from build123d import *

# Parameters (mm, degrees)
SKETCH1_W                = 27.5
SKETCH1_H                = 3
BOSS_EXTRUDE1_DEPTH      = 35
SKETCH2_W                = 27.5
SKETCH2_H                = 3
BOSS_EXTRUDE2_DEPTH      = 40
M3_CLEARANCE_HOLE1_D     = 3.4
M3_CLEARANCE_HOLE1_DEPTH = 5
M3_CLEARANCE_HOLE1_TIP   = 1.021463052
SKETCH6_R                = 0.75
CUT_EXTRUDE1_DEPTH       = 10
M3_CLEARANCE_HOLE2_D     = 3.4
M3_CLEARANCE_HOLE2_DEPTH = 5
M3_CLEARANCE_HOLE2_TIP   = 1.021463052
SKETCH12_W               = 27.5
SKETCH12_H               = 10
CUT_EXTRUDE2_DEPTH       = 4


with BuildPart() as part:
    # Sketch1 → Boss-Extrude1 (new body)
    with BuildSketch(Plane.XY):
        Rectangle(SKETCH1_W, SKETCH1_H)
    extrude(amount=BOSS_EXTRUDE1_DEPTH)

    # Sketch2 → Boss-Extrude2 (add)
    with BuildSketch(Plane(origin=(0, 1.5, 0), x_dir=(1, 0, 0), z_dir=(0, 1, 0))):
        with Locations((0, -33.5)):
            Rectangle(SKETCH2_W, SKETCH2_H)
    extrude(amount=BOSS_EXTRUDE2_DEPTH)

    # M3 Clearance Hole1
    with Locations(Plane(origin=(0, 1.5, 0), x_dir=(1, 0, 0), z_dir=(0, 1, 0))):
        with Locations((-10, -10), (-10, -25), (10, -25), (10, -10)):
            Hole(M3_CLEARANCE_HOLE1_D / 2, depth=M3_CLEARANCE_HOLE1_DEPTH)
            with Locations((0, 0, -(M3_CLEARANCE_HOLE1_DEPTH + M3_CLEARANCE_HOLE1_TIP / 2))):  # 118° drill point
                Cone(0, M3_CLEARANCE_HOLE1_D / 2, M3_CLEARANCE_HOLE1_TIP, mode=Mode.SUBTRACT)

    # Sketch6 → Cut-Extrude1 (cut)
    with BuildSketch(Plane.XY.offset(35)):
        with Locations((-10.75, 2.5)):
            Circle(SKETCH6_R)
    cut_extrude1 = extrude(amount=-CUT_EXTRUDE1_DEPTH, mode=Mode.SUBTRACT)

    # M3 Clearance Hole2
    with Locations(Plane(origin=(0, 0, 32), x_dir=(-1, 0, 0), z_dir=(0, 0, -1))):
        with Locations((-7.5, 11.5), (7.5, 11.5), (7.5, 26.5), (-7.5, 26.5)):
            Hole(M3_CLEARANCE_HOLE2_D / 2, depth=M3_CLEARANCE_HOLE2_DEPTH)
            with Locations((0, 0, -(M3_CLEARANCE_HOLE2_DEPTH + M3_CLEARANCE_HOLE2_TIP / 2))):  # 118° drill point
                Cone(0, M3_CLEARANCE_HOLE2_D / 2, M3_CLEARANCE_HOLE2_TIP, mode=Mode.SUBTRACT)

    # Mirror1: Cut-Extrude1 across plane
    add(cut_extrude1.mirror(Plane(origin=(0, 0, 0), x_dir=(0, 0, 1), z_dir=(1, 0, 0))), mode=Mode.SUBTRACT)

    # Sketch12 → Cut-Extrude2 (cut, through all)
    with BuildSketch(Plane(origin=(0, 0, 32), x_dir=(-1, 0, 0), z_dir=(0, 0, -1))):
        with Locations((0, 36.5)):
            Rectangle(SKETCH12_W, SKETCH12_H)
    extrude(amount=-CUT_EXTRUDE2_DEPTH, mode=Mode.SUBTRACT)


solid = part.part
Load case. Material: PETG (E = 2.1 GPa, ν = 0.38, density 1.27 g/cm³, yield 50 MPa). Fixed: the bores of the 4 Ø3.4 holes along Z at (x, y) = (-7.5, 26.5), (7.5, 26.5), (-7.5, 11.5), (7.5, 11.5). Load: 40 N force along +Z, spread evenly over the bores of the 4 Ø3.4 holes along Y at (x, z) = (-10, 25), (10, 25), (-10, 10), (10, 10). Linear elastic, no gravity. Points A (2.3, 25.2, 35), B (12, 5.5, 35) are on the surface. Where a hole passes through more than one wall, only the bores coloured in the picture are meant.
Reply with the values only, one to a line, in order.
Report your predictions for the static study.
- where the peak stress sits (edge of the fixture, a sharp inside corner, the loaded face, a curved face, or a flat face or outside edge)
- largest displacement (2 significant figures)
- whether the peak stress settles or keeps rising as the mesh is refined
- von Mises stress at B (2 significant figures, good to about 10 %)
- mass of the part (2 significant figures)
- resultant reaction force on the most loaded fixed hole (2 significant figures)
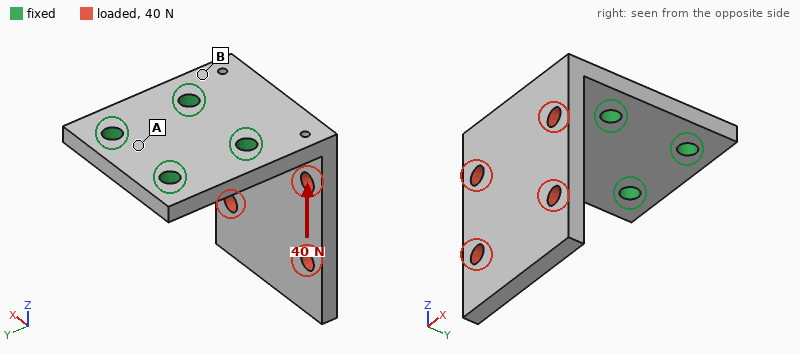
edge of the fixture
0.62 mm
keeps rising
4.9 MPa
6.5 g
23 N
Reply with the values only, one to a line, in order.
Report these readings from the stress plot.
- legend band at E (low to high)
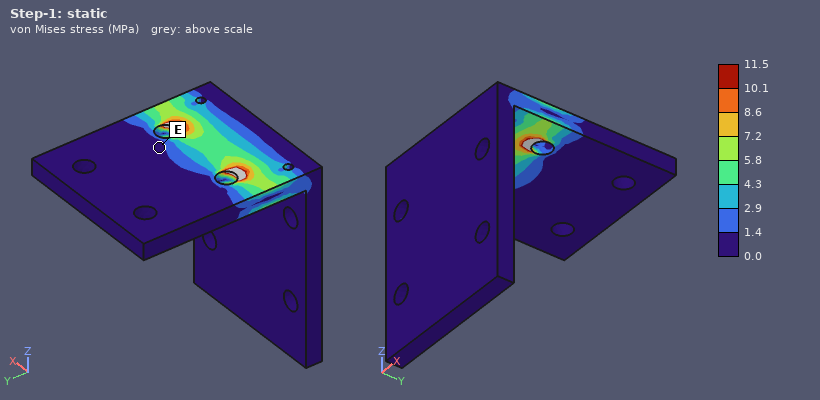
0.0 to 1.4 MPa
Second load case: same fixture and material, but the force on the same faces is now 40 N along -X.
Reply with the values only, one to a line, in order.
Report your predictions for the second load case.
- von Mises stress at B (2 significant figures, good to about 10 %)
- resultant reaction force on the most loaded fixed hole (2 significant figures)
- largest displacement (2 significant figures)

4.9 MPa
48 N
0.54 mm
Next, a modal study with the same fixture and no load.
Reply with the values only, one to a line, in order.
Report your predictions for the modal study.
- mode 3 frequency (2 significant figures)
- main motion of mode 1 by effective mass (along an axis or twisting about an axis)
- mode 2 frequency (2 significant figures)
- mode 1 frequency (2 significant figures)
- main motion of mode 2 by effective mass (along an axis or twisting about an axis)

1400 Hz
along Y
850 Hz
380 Hz
along X
